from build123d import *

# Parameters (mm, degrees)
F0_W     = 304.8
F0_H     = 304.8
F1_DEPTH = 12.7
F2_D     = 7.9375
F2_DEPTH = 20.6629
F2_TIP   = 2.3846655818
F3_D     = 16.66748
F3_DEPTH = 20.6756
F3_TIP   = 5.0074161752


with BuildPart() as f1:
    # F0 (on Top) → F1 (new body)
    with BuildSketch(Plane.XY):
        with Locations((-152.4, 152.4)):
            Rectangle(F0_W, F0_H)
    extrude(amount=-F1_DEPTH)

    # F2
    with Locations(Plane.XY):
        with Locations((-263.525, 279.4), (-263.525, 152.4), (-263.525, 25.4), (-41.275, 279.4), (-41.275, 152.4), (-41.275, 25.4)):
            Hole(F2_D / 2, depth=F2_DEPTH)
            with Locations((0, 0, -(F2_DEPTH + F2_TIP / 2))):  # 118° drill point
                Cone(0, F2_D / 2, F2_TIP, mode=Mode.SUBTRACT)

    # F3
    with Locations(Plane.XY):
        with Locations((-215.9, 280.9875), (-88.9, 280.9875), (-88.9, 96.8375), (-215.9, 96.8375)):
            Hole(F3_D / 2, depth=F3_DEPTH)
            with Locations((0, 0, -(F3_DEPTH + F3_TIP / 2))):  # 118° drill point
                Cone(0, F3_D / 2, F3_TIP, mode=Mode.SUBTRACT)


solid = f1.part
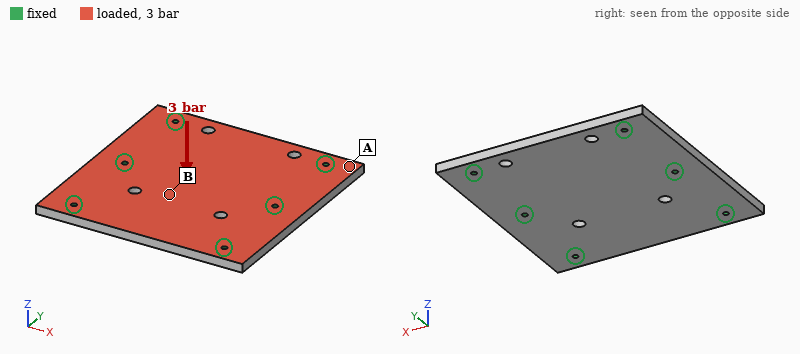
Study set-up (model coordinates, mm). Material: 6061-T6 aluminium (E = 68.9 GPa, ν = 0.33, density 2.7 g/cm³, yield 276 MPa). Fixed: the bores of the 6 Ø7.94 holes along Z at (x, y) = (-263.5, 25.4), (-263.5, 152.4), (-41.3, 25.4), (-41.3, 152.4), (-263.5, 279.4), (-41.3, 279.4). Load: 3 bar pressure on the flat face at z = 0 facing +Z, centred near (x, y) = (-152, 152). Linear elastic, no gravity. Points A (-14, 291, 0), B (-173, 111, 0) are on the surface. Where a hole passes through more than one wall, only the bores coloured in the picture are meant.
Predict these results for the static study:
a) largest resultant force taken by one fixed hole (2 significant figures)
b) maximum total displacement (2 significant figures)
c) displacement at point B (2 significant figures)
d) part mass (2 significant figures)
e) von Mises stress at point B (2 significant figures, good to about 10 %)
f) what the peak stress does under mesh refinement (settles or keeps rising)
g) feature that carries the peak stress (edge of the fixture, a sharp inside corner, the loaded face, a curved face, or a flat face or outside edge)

6.0 kN
0.24 mm
0.22 mm
3.1 kg
22 MPa
keeps rising
edge of the fixture
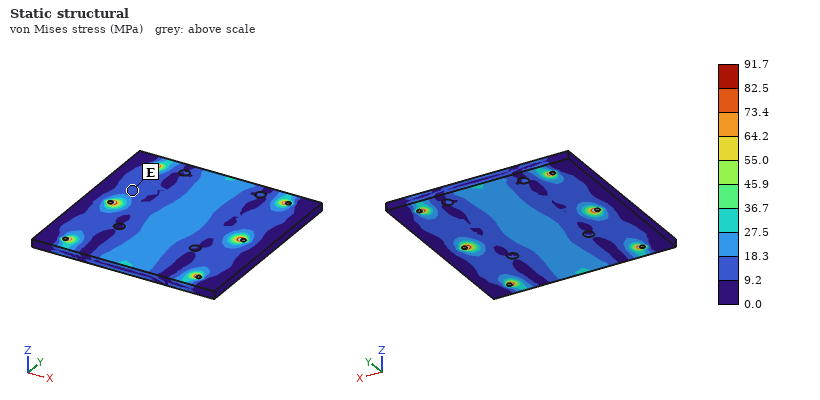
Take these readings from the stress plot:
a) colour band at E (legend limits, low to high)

9.2 to 18.3 MPa
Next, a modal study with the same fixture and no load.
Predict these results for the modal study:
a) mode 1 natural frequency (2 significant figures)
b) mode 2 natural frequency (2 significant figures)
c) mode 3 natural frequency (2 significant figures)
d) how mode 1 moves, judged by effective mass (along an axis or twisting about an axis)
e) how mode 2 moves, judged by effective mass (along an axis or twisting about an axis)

1100 Hz
1300 Hz
1900 Hz
along Z
twisting about X
